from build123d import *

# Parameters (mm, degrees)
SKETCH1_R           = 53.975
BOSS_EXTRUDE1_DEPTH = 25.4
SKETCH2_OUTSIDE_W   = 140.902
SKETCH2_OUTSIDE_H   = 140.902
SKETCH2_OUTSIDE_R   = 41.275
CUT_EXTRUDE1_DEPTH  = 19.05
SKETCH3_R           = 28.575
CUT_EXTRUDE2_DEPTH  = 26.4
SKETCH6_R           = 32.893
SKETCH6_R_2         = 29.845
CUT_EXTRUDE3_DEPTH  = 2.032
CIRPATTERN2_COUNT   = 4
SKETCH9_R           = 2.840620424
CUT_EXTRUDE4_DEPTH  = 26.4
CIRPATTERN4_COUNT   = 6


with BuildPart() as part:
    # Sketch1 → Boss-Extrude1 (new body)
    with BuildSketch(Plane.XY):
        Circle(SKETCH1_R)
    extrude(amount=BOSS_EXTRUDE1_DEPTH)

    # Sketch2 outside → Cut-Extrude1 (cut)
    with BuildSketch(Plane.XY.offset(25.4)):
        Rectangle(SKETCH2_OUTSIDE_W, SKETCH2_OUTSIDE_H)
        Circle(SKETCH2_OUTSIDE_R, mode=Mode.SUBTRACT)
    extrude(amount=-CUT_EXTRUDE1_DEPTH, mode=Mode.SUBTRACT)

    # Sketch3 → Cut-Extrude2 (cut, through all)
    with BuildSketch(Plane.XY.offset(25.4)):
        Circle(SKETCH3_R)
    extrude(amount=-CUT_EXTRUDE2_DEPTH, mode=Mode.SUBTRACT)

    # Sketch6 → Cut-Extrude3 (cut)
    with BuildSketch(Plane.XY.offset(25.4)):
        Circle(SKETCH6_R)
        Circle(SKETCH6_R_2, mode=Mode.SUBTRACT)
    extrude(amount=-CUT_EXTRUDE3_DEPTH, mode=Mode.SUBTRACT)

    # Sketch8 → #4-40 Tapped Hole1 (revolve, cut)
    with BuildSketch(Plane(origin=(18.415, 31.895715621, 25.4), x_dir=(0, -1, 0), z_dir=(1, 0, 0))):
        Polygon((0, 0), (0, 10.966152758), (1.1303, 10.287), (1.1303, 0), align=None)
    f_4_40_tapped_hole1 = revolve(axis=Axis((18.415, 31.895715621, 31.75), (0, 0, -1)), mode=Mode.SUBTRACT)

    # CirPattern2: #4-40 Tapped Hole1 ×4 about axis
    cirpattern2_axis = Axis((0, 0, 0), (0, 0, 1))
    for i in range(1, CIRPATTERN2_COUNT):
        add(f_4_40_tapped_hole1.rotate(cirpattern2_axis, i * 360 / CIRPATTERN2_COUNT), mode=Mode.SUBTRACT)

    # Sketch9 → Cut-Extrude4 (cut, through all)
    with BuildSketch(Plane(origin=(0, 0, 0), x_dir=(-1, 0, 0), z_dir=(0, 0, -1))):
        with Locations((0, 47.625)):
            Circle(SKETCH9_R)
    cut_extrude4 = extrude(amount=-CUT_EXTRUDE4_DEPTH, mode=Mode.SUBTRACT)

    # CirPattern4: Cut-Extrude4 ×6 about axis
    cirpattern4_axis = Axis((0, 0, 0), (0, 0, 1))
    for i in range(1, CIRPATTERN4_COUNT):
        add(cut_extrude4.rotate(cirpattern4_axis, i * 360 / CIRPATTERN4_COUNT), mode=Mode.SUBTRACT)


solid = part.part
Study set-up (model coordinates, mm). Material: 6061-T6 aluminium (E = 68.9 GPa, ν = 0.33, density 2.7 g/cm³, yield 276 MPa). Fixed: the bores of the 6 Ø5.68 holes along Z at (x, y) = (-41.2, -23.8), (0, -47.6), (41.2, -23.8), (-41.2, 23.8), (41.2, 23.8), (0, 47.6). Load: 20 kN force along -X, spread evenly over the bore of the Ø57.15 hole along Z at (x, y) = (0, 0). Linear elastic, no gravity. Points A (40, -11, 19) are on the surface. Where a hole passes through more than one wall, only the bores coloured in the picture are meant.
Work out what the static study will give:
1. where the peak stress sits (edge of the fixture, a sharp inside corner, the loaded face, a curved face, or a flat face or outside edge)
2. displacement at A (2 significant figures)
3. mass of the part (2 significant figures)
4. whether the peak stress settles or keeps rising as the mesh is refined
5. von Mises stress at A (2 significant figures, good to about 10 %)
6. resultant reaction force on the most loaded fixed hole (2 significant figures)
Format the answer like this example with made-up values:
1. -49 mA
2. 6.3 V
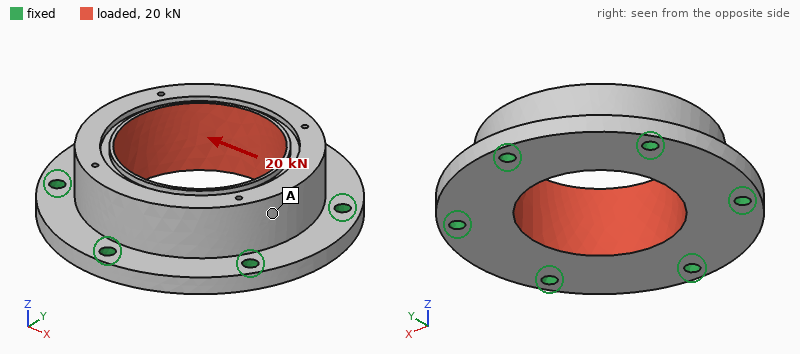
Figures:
1. edge of the fixture
2. 14 µm
3. 250 g
4. keeps rising
5. 8.4 MPa
6. 3.7 kN
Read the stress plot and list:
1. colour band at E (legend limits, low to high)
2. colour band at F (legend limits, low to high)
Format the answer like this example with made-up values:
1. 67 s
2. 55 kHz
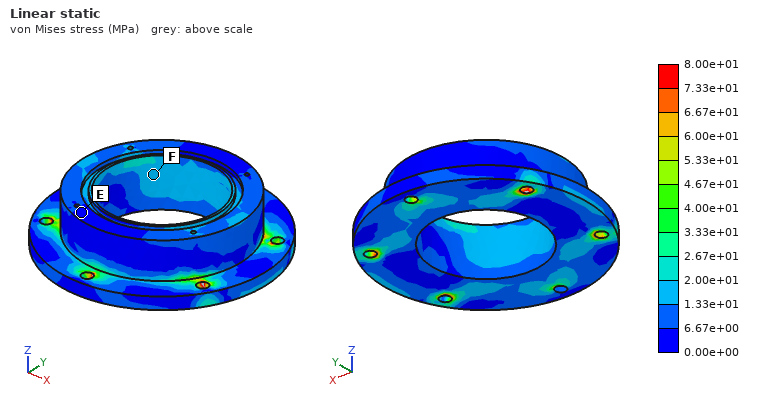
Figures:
1. 0.00e+00 to 6.67e+00 MPa
2. 1.33e+01 to 2.00e+01 MPa
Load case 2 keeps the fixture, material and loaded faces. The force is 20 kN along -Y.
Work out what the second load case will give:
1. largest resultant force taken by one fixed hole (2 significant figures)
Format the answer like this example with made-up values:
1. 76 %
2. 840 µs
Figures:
1. 4.0 kN
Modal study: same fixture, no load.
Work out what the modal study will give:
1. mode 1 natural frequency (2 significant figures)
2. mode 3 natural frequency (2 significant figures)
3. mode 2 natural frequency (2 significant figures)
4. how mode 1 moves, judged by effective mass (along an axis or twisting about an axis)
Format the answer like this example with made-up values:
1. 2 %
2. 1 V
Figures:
1. 11 kHz
2. 13 kHz
3. 13 kHz
4. along Z
